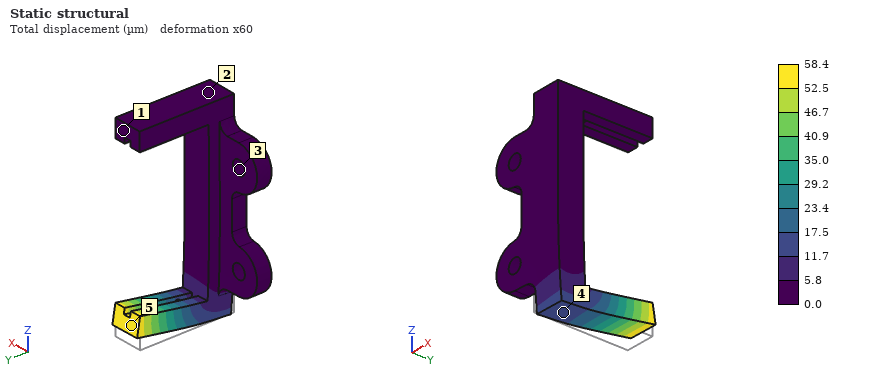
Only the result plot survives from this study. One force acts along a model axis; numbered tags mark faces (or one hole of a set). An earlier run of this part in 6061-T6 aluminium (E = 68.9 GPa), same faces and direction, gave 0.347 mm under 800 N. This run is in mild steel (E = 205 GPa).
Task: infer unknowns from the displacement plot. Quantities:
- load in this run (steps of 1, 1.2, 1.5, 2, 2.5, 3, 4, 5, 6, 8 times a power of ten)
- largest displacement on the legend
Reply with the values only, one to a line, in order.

400 N
58.4 µm
